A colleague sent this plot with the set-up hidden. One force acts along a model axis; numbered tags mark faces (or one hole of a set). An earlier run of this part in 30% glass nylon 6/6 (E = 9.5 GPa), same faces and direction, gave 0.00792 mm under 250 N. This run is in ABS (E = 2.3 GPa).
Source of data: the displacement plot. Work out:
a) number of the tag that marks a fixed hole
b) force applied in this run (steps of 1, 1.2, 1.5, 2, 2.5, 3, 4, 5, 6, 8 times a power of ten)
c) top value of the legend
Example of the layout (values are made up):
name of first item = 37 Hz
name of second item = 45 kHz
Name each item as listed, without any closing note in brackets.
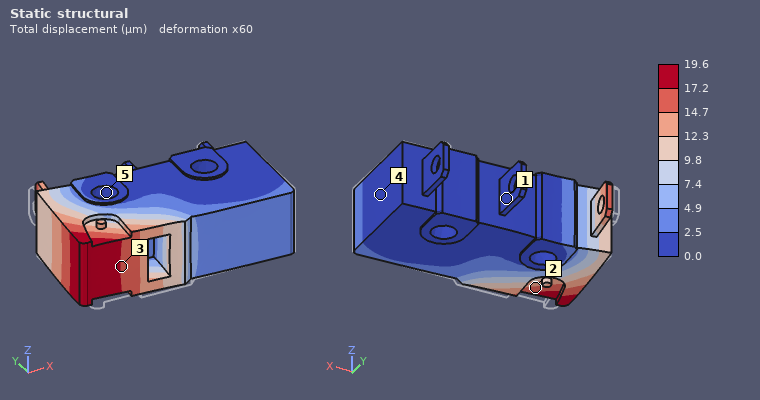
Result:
number of the tag that marks a fixed hole = 5
force applied in this run = 150 N
top value of the legend = 19.6 µm
